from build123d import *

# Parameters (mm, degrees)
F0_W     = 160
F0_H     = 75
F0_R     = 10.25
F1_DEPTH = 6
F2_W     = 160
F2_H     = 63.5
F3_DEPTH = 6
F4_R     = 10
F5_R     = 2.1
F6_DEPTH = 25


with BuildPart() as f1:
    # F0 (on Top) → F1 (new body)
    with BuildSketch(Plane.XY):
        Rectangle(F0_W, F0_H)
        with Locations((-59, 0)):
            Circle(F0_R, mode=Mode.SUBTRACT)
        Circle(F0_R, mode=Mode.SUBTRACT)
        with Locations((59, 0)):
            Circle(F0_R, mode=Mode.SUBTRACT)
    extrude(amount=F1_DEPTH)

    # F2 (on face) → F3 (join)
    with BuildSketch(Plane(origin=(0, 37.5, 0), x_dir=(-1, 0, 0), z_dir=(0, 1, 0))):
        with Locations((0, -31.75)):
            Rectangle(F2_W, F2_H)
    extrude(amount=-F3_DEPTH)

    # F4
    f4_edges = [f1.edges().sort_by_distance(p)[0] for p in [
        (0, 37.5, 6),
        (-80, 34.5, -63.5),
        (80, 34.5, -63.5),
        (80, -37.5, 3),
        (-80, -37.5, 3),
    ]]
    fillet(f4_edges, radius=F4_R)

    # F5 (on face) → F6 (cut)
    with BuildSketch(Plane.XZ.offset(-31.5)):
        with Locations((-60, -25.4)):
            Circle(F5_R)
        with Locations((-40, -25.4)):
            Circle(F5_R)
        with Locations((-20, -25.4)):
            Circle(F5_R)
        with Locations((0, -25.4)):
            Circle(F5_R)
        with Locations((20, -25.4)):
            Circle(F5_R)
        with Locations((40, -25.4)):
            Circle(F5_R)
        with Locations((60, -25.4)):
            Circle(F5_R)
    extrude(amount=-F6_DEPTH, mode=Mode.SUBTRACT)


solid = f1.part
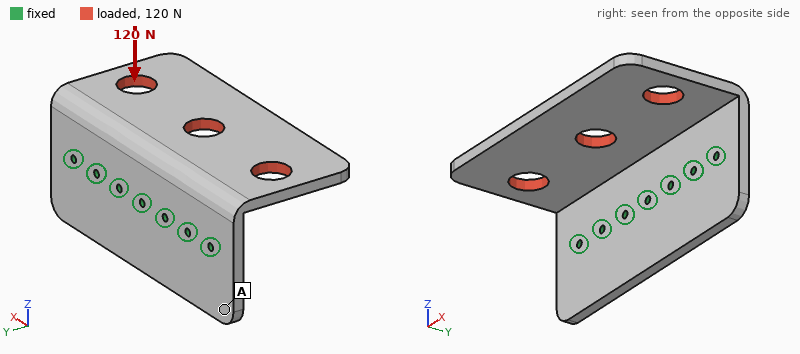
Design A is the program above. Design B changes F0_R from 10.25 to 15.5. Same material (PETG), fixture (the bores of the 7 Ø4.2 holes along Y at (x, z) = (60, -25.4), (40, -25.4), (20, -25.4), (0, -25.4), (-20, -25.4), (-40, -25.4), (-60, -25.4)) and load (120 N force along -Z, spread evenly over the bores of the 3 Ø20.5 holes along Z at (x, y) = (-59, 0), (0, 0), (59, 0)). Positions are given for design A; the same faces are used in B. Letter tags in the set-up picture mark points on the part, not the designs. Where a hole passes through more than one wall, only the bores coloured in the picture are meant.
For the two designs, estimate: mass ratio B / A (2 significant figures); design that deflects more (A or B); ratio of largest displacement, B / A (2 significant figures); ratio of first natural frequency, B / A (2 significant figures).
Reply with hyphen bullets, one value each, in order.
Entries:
- 0.94
- B
- 1.1
- 0.99
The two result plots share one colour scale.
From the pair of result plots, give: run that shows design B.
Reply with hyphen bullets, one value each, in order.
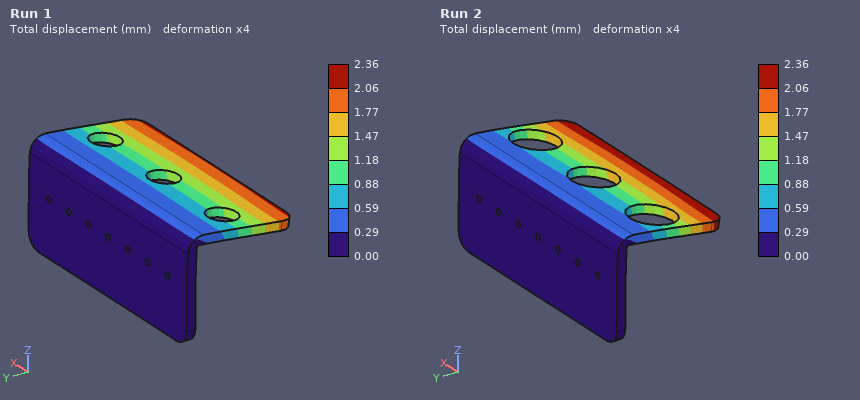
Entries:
- Run 2
